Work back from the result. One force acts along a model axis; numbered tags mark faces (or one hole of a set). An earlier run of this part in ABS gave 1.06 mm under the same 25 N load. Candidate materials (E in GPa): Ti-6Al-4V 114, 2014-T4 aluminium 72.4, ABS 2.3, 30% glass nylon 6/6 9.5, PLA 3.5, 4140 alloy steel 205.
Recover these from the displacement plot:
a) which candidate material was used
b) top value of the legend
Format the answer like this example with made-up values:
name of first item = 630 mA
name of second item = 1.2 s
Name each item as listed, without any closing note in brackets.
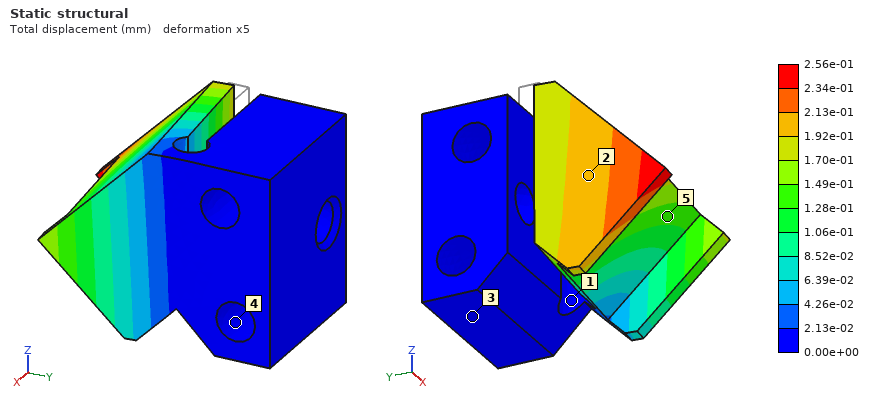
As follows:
which candidate material was used = 30% glass nylon 6/6
top value of the legend = 2.56e-01 mm
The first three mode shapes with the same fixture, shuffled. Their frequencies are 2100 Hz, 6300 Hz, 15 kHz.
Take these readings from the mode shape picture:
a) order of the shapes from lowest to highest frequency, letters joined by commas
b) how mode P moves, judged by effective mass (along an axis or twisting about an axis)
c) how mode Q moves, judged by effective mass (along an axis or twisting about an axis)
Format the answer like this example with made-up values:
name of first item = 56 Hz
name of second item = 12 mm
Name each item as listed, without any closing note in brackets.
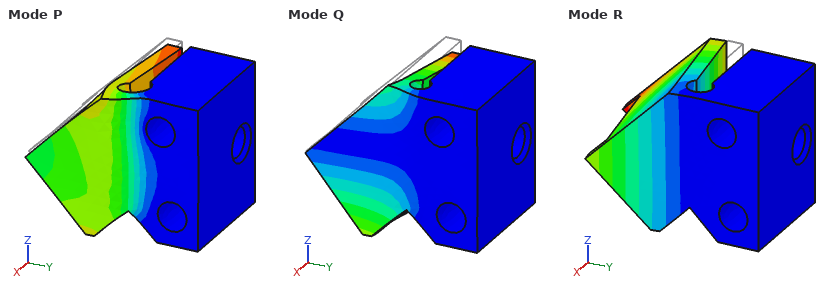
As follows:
order of the shapes from lowest to highest frequency, letters joined by commas = R, Q, P
how mode P moves, judged by effective mass = along X
how mode Q moves, judged by effective mass = along Z
